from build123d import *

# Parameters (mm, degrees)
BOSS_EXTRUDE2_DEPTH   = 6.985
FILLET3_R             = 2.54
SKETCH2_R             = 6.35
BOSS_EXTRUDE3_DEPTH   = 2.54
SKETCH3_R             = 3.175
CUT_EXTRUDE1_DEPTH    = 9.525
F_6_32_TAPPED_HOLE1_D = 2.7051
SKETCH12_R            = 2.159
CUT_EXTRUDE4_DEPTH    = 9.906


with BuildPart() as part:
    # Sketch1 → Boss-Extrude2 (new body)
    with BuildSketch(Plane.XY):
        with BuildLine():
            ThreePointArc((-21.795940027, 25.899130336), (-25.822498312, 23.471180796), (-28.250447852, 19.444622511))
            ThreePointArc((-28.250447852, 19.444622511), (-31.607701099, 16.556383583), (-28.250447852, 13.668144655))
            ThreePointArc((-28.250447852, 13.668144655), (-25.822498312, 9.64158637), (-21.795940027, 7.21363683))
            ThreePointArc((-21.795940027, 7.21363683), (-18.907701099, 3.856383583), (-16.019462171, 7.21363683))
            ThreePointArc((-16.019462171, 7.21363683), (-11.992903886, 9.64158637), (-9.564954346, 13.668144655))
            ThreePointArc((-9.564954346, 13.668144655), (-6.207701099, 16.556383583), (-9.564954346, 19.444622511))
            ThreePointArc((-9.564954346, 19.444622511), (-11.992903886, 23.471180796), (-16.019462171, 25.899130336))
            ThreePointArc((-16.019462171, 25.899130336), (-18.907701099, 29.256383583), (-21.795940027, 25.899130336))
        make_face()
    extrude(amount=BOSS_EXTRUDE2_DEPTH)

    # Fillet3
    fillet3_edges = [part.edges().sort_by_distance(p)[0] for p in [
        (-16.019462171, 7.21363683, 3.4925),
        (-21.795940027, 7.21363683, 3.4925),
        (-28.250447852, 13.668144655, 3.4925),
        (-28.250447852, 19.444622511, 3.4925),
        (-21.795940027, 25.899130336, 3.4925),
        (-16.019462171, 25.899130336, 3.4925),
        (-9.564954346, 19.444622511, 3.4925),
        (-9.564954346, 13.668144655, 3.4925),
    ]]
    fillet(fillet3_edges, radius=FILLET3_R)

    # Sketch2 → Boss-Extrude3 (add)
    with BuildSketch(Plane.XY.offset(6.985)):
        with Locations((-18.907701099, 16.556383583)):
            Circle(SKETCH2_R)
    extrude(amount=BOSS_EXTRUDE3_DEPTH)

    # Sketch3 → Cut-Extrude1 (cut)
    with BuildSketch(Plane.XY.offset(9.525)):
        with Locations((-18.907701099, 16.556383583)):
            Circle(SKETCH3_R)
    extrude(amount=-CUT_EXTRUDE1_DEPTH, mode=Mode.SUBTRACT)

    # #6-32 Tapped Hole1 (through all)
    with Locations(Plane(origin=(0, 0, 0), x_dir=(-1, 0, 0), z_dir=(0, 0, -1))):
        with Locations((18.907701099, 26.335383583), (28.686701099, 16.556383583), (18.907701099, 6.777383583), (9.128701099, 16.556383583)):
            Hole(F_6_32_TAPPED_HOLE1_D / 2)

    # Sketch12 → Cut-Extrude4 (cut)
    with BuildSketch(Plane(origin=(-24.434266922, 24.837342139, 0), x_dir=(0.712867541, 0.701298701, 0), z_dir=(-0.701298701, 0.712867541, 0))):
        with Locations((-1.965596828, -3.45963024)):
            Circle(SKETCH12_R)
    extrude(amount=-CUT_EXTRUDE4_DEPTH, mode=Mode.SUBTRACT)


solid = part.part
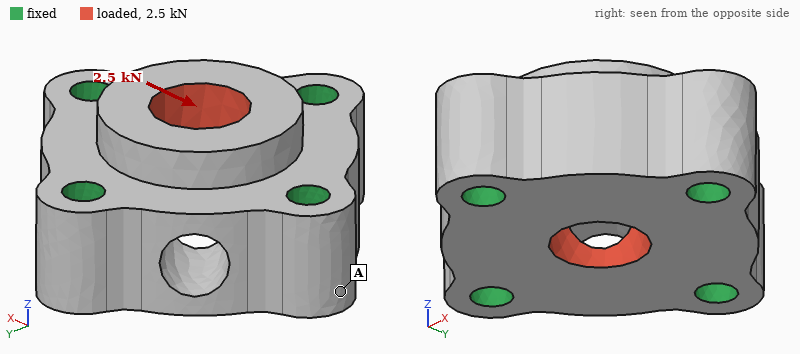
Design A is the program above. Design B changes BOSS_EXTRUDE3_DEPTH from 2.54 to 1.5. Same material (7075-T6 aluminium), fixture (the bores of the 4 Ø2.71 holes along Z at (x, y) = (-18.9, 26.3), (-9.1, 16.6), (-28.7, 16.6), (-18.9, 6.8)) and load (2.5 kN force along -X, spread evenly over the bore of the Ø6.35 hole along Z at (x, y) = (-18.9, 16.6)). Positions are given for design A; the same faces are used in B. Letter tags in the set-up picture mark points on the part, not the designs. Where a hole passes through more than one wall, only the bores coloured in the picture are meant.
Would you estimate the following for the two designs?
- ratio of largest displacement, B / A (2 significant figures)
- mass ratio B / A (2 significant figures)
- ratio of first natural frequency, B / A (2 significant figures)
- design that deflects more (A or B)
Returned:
0.83
0.96
1.0
A
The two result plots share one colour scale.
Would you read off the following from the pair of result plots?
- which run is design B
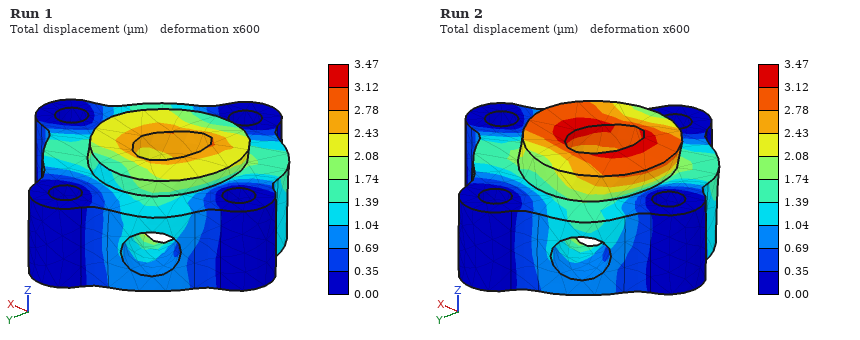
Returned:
Run 1
